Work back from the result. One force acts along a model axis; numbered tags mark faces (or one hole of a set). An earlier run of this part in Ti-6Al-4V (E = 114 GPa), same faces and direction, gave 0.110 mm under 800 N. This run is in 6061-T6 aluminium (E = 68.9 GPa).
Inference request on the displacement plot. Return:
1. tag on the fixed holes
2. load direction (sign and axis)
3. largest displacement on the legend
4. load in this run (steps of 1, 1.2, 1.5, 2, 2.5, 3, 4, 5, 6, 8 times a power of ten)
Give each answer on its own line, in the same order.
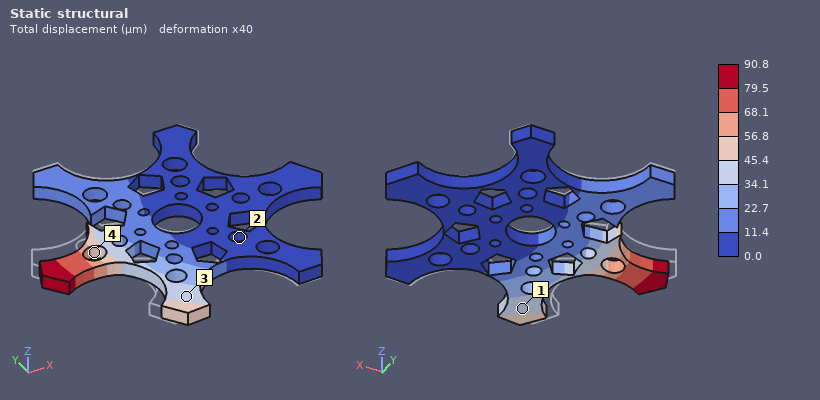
2
-Y
90.8 µm
400 N
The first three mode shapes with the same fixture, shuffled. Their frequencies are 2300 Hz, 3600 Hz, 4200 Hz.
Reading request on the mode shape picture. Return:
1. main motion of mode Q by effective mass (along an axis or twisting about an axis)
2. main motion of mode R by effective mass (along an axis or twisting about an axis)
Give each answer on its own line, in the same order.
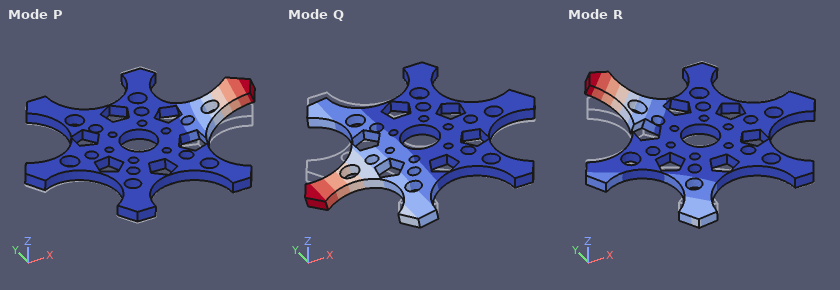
along Z
twisting about X
